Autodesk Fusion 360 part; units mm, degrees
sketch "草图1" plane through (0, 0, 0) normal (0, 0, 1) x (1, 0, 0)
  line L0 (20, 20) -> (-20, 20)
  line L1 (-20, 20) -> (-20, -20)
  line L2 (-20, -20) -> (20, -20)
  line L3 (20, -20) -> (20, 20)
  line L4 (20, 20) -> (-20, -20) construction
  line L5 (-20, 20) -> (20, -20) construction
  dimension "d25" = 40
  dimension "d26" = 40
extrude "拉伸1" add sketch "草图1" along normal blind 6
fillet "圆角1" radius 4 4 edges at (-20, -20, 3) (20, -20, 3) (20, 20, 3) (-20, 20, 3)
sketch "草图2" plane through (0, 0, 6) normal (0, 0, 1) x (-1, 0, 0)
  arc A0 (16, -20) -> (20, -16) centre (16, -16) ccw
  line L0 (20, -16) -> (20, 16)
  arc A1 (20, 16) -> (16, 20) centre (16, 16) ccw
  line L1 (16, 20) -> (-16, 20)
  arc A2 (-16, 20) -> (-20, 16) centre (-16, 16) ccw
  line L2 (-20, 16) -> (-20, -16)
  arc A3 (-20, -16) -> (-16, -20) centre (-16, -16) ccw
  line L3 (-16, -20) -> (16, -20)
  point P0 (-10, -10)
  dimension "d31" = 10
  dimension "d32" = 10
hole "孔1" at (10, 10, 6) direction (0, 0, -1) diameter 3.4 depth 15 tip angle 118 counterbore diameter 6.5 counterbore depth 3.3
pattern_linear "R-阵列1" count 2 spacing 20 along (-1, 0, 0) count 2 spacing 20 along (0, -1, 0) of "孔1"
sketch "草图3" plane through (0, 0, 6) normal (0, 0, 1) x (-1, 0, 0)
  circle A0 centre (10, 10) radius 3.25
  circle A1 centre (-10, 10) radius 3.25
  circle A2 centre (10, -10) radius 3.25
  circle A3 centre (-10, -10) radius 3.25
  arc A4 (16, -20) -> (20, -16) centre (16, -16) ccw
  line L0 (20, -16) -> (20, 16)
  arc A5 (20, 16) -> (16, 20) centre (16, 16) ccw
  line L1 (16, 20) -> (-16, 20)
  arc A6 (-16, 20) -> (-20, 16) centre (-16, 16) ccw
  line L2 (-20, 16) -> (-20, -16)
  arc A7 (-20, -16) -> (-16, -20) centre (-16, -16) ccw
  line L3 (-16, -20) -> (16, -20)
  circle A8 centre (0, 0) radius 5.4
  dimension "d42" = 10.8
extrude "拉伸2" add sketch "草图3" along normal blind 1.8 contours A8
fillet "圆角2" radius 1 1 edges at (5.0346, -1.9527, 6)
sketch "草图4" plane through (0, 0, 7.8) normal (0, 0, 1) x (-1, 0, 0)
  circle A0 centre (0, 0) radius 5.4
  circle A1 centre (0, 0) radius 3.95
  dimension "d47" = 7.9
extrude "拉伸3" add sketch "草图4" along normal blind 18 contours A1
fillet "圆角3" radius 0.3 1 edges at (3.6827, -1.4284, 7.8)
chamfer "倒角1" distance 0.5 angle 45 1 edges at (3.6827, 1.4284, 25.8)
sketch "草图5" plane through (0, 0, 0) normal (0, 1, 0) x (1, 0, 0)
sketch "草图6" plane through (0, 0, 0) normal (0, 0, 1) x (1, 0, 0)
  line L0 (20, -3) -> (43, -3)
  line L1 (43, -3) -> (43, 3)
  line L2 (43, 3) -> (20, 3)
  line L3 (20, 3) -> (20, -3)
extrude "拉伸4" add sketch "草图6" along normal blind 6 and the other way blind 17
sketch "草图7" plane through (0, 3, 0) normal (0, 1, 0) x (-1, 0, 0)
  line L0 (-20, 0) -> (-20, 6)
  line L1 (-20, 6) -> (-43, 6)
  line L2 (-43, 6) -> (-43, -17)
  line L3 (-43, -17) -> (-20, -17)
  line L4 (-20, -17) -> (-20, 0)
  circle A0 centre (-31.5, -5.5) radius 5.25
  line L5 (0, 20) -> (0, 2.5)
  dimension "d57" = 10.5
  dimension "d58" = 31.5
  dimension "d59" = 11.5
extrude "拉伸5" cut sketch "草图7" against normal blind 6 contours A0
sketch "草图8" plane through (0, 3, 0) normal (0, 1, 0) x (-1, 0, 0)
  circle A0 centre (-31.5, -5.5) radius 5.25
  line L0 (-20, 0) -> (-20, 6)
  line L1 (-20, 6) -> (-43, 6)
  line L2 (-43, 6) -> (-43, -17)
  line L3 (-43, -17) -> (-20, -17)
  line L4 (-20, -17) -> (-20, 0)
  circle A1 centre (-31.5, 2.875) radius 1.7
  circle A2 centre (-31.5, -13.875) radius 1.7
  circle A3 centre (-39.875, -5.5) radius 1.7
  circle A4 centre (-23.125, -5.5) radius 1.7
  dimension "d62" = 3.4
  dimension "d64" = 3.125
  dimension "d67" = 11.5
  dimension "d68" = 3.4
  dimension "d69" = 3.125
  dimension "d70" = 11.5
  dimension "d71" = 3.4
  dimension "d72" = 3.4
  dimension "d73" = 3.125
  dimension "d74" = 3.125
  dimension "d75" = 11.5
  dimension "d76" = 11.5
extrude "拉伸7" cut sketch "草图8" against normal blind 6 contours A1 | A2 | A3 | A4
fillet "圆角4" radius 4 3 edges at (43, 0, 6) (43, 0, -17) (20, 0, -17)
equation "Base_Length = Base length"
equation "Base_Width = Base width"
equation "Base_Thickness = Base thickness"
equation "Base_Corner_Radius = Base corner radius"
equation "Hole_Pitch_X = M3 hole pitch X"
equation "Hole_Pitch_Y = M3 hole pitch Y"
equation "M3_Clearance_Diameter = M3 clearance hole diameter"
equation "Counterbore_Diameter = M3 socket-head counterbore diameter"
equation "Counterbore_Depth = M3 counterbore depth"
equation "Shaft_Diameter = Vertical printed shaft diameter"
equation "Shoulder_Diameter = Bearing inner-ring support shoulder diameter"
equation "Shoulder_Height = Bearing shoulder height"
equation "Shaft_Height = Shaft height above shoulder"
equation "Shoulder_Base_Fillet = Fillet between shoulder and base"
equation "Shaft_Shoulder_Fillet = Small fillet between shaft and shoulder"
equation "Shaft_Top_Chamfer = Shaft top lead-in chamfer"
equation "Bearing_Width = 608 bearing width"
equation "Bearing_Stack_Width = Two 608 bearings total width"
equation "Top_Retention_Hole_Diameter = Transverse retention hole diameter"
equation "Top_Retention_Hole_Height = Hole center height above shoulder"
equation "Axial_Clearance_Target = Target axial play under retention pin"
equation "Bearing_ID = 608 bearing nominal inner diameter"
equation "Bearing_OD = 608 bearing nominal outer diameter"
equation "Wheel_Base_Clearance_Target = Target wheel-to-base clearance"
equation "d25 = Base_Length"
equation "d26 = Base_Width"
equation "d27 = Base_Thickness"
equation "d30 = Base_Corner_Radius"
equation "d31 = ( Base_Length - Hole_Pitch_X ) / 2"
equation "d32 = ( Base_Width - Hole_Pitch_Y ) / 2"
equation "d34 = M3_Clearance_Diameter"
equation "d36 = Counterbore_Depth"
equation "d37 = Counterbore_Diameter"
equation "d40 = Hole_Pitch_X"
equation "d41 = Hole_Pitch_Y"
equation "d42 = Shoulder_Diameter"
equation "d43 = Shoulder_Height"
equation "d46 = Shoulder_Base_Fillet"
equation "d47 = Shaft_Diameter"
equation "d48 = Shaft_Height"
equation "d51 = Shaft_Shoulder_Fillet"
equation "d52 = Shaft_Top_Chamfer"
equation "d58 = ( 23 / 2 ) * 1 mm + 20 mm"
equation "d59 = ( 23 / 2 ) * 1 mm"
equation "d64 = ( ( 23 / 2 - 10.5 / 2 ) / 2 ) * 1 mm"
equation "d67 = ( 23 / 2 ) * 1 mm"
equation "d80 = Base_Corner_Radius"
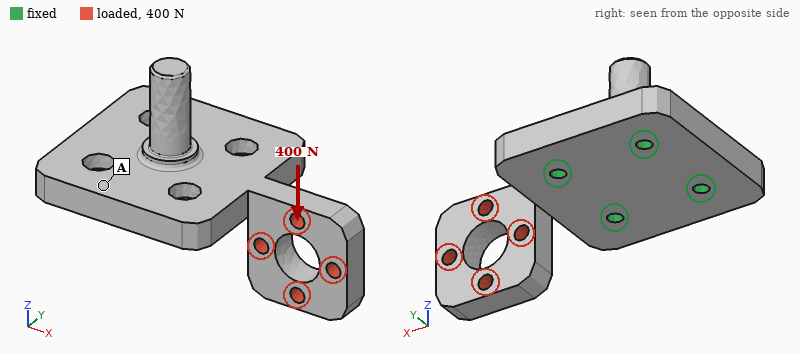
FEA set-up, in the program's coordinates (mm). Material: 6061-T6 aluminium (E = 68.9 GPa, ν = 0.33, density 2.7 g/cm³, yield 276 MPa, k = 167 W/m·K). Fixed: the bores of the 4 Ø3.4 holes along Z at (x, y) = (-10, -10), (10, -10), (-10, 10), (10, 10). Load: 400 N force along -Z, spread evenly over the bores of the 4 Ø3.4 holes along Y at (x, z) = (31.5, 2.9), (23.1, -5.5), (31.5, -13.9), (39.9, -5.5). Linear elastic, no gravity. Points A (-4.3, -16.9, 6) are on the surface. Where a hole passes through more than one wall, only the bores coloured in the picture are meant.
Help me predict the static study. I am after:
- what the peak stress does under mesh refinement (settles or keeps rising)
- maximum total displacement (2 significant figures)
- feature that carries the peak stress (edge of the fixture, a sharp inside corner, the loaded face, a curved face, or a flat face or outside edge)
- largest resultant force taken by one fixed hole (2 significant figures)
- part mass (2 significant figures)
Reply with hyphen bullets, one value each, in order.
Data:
- keeps rising
- 0.22 mm
- edge of the fixture
- 500 N
- 34 g
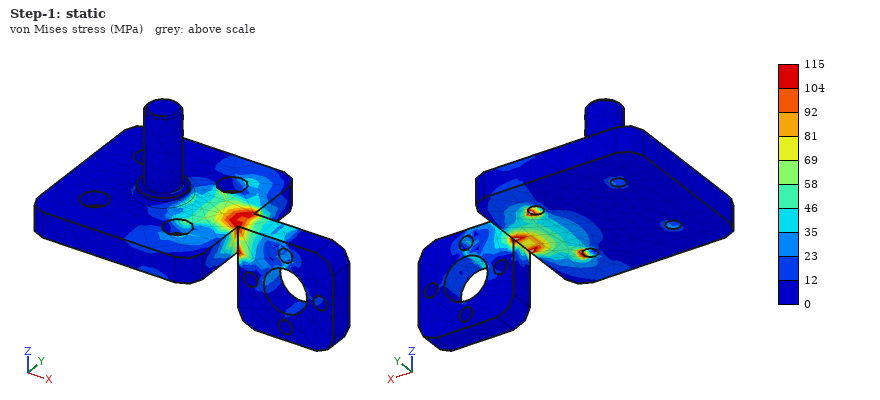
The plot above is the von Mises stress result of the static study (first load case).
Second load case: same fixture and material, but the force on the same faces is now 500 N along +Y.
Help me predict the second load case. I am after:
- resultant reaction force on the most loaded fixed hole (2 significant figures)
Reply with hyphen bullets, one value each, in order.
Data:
- 470 N
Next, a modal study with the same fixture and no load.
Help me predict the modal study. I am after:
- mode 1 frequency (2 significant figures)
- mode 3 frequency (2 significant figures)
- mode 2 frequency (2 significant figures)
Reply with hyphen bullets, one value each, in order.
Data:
- 2900 Hz
- 7400 Hz
- 3700 Hz
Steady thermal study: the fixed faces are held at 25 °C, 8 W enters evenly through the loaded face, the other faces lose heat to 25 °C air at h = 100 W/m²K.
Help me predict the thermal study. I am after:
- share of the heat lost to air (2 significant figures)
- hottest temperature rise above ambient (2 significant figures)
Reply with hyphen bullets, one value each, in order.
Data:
- 27 %
- 16 K
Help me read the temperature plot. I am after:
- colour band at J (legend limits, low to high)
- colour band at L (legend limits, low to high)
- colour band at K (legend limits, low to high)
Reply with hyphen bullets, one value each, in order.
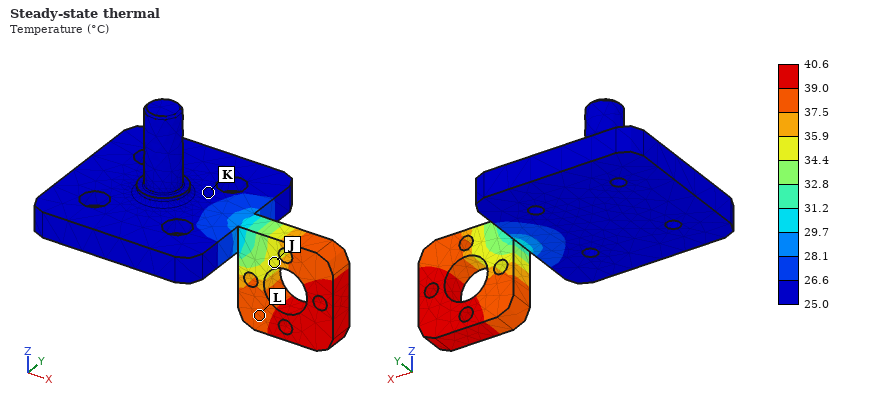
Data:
- 34.4 to 35.9 °C
- 37.5 to 39.0 °C
- 25.0 to 26.6 °C
